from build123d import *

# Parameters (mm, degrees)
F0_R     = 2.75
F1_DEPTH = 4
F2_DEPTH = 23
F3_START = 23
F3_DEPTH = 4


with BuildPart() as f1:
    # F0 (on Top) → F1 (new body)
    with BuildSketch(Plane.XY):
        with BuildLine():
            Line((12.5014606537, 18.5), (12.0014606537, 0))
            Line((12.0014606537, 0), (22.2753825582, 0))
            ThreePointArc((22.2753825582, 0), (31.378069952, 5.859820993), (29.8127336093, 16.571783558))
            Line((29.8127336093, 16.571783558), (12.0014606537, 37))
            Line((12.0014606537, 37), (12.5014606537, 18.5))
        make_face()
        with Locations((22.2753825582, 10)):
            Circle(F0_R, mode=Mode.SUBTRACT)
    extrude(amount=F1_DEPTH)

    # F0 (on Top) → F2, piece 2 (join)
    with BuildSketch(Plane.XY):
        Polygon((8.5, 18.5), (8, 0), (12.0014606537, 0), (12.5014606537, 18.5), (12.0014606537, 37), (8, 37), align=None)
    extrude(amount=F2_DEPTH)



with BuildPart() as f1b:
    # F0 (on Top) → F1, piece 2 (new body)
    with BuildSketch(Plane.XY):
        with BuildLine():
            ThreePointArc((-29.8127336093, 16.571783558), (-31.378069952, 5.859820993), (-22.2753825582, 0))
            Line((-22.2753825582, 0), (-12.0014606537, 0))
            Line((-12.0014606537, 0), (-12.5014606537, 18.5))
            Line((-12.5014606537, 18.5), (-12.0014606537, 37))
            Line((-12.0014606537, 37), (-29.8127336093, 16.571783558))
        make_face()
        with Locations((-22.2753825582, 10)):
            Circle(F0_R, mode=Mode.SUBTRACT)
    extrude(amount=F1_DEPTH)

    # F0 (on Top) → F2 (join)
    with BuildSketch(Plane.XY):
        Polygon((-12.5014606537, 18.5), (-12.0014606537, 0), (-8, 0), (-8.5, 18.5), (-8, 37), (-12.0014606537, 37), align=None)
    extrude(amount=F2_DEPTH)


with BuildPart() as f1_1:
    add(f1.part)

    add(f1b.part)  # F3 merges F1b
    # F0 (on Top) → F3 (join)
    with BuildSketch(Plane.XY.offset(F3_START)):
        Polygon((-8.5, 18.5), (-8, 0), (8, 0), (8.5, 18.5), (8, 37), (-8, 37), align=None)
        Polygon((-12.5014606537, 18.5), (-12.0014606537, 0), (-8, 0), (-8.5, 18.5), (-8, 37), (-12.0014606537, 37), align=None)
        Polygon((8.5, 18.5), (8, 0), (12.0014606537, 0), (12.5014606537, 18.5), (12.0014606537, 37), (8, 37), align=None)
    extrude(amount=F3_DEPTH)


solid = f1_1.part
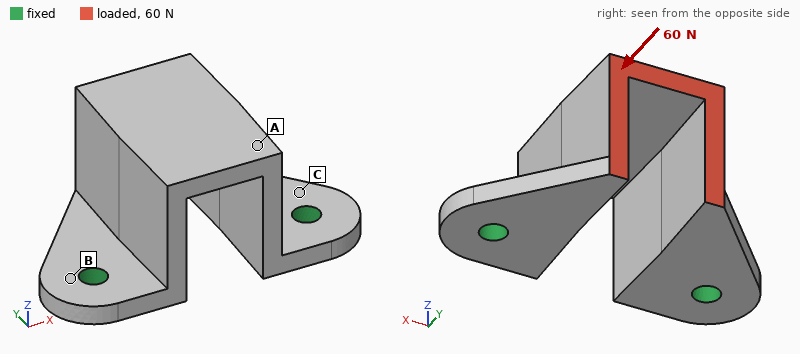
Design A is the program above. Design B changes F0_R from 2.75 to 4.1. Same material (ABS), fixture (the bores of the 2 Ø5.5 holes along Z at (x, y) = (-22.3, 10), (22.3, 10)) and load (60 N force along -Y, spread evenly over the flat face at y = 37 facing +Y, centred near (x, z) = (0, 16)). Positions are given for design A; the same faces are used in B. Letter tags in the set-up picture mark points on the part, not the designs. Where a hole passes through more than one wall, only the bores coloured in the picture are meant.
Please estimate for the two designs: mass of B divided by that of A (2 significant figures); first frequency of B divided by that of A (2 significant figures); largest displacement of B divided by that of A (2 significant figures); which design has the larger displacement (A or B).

0.98
1.2
0.70
A
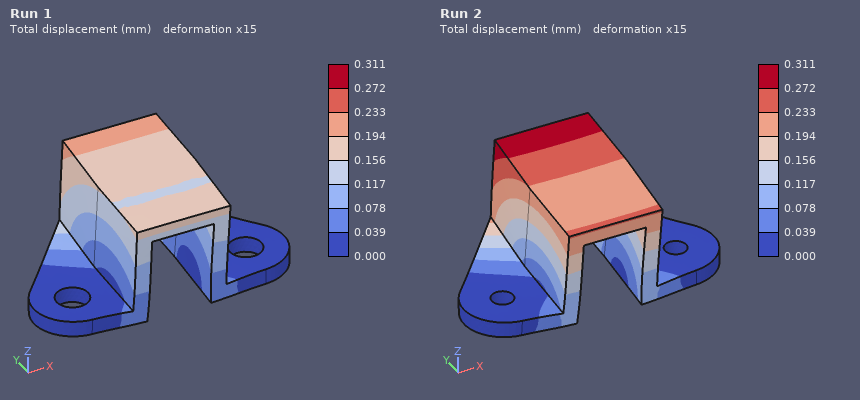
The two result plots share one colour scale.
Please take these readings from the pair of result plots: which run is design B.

Run 1
